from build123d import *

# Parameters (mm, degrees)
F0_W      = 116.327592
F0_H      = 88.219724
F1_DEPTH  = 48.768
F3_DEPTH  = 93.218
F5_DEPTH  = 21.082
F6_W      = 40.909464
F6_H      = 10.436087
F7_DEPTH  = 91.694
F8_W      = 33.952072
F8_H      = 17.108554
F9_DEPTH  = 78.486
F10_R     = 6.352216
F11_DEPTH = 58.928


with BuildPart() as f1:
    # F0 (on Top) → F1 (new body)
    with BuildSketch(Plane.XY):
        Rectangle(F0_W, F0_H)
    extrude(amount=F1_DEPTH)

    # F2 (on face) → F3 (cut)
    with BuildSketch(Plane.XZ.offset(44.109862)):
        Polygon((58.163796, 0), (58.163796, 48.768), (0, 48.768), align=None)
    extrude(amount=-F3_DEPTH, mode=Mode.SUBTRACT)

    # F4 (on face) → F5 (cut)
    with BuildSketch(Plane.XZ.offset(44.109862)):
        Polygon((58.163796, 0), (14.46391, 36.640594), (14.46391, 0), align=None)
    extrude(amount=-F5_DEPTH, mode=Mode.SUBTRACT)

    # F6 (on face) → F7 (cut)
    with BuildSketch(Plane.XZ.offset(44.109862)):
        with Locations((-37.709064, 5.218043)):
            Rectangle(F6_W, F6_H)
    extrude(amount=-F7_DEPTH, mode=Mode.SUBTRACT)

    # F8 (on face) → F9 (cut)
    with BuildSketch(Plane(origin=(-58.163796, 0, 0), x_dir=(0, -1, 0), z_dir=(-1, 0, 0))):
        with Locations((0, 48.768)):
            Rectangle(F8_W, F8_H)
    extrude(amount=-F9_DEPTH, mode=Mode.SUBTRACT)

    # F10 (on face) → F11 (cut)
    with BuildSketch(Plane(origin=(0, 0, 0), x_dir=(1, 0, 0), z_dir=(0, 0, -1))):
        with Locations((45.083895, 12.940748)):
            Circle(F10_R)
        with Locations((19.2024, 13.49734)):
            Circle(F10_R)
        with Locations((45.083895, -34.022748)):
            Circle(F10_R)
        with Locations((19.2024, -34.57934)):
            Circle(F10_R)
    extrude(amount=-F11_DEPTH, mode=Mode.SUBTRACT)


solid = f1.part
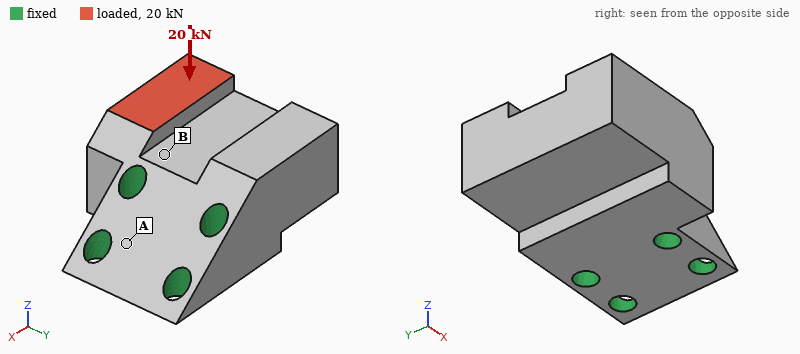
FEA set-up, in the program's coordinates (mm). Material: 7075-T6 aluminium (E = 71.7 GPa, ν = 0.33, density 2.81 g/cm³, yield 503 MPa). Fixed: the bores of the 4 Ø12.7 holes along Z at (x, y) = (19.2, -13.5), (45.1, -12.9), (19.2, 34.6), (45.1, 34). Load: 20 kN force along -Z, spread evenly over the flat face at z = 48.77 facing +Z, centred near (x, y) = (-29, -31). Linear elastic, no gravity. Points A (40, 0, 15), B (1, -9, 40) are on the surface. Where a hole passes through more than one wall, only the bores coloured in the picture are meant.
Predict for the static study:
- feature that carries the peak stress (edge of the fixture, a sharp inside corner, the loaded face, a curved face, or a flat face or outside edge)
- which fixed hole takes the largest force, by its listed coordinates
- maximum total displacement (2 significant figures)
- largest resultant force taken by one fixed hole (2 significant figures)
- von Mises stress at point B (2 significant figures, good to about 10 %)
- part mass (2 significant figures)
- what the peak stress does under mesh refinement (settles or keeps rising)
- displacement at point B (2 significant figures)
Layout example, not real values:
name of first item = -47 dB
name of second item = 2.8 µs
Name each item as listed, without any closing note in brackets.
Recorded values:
feature that carries the peak stress = edge of the fixture
which fixed hole takes the largest force, by its listed coordinates = (19.2, -13.5)
maximum total displacement = 0.15 mm
largest resultant force taken by one fixed hole = 21 kN
von Mises stress at point B = 35 MPa
part mass = 820 g
what the peak stress does under mesh refinement = keeps rising
displacement at point B = 0.025 mm
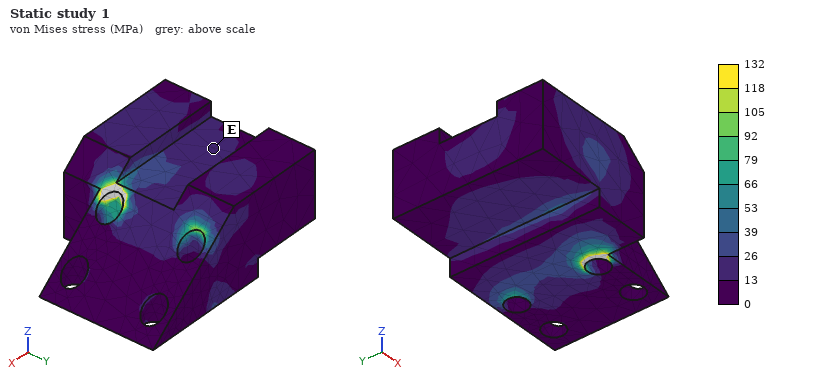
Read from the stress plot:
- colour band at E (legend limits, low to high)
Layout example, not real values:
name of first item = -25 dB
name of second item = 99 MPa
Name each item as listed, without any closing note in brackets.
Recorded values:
colour band at E = 13 to 26 MPa
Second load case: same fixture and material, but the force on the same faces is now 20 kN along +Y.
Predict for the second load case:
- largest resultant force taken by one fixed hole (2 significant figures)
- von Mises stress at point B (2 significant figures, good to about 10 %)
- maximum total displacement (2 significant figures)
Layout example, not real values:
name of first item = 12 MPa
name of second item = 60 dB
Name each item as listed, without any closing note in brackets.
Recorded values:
largest resultant force taken by one fixed hole = 21 kN
von Mises stress at point B = 47 MPa
maximum total displacement = 92 µm
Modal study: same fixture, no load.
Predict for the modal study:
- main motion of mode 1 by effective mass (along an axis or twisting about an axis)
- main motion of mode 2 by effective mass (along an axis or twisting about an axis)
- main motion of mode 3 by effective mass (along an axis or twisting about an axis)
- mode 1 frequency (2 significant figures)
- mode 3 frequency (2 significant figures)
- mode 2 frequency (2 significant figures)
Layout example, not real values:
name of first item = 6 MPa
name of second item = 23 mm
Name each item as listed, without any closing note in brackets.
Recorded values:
main motion of mode 1 by effective mass = along Z
main motion of mode 2 by effective mass = along Y
main motion of mode 3 by effective mass = twisting about X
mode 1 frequency = 4100 Hz
mode 3 frequency = 6800 Hz
mode 2 frequency = 5800 Hz
